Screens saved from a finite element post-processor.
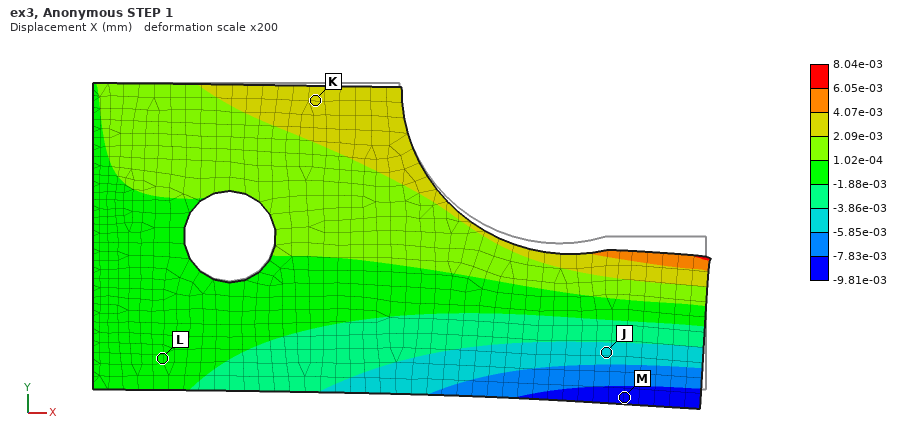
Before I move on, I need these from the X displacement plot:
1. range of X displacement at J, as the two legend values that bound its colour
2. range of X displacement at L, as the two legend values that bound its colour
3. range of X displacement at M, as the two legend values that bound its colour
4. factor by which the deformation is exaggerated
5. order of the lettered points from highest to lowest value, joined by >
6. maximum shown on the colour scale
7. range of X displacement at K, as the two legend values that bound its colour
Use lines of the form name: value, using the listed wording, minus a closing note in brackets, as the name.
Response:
range of X displacement at J, as the two legend values that bound its colour: -5.85e-03 to -3.86e-03 mm
range of X displacement at L, as the two legend values that bound its colour: -1.88e-03 to 1.02e-04 mm
range of X displacement at M, as the two legend values that bound its colour: -9.81e-03 to -7.83e-03 mm
factor by which the deformation is exaggerated: 200
order of the lettered points from highest to lowest value, joined by >: K > L > J > M
maximum shown on the colour scale: 8.04e-03 mm
range of X displacement at K, as the two legend values that bound its colour: 2.09e-03 to 4.07e-03 mm
